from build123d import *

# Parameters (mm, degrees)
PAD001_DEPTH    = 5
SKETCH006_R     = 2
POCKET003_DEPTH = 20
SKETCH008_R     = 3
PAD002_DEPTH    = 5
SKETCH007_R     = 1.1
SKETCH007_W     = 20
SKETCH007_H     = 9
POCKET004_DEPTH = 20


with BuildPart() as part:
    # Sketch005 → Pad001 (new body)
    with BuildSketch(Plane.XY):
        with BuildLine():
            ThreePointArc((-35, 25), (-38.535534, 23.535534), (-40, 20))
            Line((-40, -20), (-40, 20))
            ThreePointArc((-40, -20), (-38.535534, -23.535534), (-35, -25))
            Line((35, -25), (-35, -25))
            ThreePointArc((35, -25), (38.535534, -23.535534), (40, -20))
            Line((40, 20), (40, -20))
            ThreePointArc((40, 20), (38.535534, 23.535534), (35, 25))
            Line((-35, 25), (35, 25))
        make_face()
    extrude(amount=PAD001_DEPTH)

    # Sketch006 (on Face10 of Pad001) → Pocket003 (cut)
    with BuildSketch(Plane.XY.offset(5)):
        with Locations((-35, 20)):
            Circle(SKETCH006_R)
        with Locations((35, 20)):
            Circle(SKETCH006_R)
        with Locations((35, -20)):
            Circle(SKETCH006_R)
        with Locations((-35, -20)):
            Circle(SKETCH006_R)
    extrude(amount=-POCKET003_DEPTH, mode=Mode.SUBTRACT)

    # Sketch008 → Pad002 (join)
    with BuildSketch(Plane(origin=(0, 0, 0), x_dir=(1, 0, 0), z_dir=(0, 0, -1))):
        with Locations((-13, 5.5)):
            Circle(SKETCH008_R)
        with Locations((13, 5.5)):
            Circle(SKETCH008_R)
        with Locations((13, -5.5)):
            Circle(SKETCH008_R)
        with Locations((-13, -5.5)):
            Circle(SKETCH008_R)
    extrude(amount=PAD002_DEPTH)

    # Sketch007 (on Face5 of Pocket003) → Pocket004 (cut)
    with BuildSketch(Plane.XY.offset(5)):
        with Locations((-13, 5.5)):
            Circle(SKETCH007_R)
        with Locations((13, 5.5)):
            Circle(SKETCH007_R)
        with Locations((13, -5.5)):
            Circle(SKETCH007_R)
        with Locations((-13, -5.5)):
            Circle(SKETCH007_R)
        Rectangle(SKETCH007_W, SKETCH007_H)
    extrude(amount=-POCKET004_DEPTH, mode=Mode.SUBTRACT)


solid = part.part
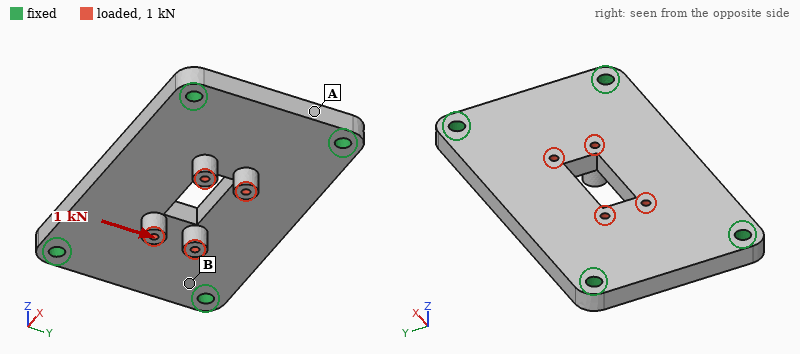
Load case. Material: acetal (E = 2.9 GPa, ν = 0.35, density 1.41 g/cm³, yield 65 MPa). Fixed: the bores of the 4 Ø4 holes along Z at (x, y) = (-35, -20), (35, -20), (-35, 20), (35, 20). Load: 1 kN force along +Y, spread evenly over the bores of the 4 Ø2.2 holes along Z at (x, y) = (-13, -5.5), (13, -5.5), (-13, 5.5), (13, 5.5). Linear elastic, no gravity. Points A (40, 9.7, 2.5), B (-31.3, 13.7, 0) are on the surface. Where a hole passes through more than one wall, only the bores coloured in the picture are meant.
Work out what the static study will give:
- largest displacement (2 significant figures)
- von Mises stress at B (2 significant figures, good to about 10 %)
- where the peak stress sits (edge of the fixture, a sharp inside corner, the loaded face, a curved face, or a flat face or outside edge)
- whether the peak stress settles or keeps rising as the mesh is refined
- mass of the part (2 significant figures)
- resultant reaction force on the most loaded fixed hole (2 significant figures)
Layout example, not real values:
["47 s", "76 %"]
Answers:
["0.16 mm", "6.0 MPa", "edge of the fixture", "keeps rising", "27 g", "310 N"]
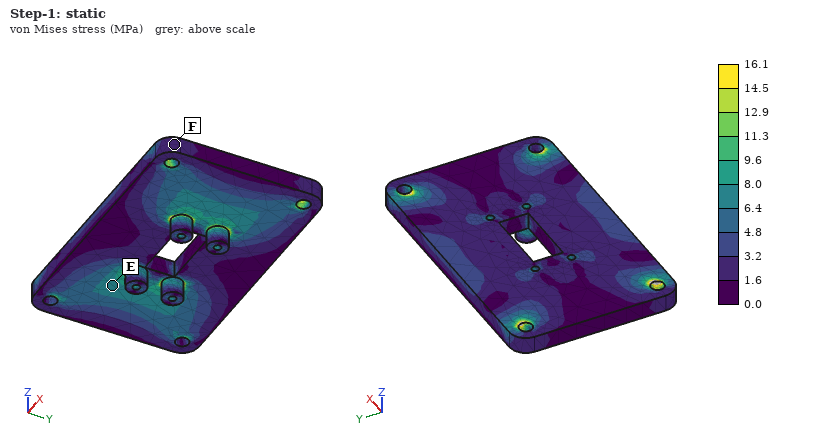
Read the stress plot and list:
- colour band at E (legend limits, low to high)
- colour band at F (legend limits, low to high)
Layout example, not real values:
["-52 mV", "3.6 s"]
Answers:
["6.4 to 8.0 MPa", "1.6 to 3.2 MPa"]
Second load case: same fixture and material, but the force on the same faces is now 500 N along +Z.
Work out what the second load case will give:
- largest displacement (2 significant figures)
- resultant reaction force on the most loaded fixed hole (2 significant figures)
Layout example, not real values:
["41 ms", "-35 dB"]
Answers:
["0.81 mm", "130 N"]
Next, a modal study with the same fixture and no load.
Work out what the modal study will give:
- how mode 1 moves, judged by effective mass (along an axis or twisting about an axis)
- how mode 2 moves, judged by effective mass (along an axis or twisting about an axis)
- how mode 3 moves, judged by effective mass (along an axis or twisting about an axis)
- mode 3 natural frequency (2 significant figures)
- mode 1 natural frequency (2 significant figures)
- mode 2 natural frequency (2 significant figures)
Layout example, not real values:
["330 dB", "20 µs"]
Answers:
["along Z", "twisting about X", "twisting about Y", "3100 Hz", "1300 Hz", "1900 Hz"]
